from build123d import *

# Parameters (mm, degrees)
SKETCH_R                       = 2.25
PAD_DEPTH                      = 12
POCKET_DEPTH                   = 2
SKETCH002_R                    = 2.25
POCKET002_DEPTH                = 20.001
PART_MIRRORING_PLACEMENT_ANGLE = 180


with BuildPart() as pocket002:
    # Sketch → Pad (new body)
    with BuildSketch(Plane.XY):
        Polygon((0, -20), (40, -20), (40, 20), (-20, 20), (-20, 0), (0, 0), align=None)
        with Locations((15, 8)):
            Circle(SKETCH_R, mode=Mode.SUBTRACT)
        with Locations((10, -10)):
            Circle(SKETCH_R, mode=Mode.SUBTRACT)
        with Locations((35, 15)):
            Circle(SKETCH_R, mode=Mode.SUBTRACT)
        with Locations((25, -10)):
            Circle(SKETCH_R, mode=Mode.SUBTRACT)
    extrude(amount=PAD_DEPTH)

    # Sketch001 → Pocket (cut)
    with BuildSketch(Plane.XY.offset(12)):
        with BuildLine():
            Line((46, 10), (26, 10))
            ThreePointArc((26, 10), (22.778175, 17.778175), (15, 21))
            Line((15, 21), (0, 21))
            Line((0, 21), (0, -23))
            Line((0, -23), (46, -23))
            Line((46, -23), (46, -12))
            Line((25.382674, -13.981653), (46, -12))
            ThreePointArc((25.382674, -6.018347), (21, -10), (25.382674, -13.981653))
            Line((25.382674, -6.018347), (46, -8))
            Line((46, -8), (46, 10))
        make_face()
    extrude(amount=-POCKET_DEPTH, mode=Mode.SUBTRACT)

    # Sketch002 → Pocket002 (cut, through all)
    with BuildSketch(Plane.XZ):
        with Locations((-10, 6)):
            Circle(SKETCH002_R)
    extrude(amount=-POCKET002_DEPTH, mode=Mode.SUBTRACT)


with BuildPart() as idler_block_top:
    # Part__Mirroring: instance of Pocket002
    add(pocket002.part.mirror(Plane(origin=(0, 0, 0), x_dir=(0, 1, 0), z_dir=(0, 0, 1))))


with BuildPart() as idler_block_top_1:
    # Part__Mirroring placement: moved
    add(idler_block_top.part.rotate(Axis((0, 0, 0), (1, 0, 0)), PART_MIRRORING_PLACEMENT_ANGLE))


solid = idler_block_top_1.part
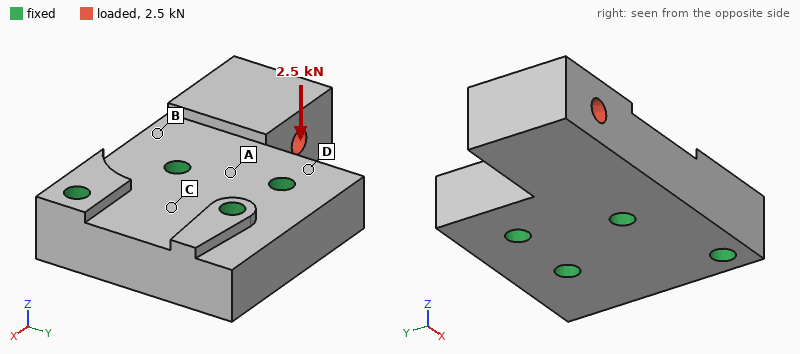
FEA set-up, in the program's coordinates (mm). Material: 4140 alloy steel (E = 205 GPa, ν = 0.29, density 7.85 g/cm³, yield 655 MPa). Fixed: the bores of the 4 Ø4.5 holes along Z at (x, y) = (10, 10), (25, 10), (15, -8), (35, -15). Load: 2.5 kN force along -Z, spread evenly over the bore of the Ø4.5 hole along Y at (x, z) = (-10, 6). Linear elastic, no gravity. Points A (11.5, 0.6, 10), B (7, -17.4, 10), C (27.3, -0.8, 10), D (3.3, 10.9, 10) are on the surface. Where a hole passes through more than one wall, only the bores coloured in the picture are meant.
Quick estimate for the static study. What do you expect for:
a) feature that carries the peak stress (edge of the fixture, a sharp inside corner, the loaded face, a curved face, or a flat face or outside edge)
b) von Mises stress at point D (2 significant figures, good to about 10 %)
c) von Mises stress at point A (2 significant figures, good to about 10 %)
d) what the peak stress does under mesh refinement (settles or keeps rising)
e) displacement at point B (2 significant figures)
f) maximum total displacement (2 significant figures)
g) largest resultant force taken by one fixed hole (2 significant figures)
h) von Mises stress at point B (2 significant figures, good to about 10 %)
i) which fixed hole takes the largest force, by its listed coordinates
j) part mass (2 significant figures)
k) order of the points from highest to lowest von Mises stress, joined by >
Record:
edge of the fixture
33 MPa
62 MPa
keeps rising
8.7 µm
56 µm
2.4 kN
83 MPa
(15, -8)
160 g
B > A > D > C
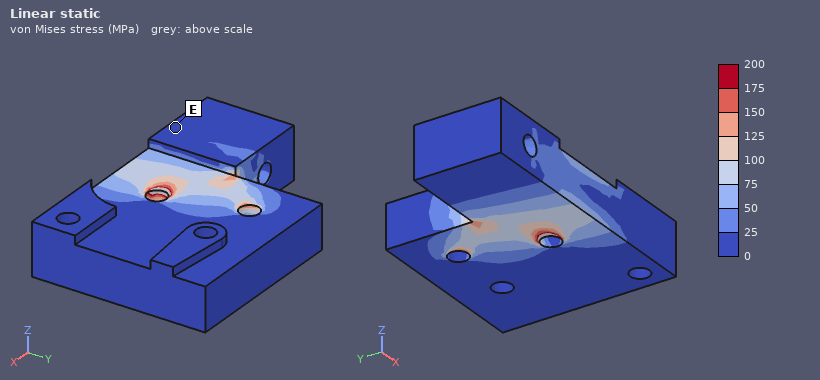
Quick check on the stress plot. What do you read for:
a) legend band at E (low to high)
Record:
0 to 25 MPa
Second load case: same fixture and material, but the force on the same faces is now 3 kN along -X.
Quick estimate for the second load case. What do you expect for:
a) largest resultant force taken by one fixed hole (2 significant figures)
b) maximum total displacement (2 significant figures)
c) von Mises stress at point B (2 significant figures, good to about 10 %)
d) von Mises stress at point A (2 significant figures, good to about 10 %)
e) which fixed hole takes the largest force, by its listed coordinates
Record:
2.2 kN
5.0 µm
20 MPa
7.2 MPa
(15, -8)
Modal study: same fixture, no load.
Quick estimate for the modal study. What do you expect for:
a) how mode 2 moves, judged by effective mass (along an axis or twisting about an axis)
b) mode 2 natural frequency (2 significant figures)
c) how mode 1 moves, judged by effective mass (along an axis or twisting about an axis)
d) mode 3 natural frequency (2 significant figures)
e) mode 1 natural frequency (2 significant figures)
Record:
along Y
14 kHz
along Z
19 kHz
6800 Hz
